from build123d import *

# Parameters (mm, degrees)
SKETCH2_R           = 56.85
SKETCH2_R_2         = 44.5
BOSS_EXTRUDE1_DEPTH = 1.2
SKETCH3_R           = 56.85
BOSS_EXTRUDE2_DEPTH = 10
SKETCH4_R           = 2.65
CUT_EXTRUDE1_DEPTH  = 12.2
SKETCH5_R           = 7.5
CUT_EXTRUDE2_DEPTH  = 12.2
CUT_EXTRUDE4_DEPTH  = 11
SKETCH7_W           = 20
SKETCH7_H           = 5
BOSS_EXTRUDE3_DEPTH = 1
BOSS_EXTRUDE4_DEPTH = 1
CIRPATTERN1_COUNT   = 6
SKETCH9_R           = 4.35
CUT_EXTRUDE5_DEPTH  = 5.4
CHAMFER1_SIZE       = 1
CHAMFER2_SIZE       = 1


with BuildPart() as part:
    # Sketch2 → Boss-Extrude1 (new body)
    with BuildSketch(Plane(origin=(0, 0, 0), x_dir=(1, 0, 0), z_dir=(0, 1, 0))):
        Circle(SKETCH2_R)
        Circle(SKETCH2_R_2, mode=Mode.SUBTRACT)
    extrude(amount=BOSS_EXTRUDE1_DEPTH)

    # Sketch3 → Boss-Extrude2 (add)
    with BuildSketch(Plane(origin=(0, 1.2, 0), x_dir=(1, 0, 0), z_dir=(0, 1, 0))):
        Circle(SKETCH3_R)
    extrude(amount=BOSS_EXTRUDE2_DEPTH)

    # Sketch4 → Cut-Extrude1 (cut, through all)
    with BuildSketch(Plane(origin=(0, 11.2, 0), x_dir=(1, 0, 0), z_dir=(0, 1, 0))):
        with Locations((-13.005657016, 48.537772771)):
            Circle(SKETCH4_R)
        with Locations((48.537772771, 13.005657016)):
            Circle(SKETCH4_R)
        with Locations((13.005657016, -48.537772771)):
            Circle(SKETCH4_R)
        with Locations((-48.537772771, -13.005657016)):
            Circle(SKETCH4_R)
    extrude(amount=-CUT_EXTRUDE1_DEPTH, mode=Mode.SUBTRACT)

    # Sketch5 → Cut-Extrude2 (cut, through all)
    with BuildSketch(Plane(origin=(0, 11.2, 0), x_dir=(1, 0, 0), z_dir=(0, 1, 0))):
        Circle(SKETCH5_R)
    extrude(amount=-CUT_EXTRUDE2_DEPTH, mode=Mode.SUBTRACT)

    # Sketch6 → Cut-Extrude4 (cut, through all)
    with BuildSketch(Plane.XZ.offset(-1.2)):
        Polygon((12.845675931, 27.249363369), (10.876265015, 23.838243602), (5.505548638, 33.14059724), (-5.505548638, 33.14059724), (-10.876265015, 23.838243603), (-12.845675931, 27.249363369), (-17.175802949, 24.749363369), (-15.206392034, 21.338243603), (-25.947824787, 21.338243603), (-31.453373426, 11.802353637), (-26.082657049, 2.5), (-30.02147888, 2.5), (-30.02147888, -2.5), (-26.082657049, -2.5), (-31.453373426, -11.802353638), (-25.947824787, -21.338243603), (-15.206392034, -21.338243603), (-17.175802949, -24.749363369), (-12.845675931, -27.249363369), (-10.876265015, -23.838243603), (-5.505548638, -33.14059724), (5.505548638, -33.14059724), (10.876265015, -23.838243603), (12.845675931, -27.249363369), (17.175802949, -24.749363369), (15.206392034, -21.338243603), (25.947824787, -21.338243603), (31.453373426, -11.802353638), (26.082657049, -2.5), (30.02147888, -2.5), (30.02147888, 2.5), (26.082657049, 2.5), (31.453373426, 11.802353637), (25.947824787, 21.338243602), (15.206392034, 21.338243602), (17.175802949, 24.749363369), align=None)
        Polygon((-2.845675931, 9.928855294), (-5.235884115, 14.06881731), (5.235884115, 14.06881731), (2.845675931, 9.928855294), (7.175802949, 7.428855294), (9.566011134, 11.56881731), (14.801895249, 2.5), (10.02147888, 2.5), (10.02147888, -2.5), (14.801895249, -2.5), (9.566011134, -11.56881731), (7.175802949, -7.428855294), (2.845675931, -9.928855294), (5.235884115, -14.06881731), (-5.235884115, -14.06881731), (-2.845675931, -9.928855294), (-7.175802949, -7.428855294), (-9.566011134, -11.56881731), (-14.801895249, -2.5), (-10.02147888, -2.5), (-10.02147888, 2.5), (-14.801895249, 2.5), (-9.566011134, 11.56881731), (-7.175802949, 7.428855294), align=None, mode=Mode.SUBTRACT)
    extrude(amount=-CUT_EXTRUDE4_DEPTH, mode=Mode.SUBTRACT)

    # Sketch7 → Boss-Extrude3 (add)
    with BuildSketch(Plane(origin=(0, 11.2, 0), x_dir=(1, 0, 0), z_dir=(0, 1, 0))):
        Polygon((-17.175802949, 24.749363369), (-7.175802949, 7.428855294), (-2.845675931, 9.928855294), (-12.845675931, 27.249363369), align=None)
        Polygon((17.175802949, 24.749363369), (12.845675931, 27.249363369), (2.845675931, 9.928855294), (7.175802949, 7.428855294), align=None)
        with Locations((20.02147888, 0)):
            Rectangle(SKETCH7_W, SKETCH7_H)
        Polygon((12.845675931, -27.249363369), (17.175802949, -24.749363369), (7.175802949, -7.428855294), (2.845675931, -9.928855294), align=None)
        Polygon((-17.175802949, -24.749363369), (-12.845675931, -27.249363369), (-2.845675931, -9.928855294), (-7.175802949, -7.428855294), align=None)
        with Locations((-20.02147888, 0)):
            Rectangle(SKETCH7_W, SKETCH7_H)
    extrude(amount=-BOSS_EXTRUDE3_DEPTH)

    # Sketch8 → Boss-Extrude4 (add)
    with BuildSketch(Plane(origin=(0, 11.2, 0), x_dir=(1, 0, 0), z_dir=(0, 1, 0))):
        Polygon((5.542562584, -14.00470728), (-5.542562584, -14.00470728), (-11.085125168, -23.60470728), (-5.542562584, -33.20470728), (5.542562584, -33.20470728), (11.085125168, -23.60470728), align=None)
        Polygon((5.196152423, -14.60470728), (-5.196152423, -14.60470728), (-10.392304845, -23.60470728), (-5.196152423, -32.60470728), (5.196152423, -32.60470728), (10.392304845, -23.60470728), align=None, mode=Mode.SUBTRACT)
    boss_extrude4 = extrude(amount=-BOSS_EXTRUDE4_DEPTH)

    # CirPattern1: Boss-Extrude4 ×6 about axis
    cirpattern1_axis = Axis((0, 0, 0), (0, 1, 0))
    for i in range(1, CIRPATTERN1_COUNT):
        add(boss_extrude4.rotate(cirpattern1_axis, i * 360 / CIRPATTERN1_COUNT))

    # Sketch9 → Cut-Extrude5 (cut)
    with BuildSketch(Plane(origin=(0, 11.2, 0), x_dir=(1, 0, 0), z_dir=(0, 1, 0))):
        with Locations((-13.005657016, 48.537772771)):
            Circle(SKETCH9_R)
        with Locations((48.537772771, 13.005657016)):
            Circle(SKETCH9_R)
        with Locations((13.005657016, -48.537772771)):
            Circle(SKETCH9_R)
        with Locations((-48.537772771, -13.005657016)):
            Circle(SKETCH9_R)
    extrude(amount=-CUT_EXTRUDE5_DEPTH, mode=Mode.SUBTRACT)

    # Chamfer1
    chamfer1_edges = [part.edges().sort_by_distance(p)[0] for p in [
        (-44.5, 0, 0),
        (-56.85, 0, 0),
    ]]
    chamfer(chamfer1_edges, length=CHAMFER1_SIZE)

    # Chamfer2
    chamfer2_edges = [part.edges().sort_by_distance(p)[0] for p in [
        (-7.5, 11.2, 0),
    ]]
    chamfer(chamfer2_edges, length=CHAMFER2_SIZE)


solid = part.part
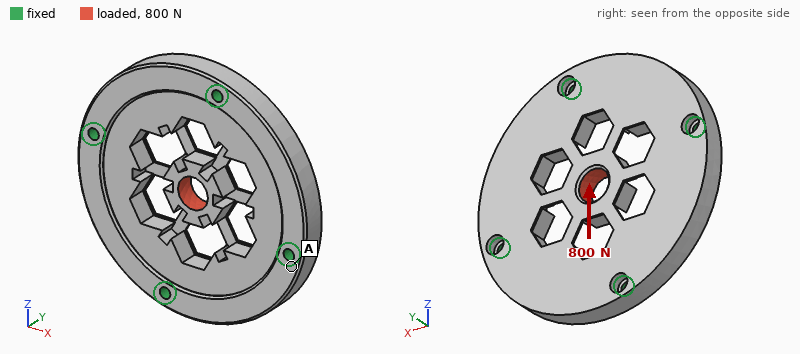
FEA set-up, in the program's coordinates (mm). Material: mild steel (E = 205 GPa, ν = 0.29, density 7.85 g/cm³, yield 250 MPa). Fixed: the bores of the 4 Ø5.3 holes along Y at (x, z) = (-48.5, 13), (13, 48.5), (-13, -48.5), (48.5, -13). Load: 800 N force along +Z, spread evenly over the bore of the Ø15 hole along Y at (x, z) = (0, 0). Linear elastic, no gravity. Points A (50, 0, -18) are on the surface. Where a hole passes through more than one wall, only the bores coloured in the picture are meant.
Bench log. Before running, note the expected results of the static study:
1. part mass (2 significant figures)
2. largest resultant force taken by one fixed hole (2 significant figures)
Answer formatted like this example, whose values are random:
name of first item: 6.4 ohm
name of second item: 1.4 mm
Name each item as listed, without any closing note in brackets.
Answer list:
part mass: 620 g
largest resultant force taken by one fixed hole: 230 N
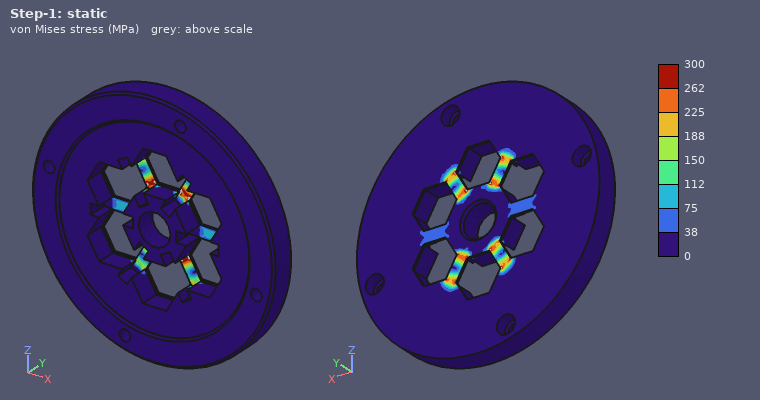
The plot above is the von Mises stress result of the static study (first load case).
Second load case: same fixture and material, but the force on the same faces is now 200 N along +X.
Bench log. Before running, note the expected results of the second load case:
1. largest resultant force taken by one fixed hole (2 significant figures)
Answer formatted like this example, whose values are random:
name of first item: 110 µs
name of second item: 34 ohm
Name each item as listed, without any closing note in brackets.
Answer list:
largest resultant force taken by one fixed hole: 58 N
